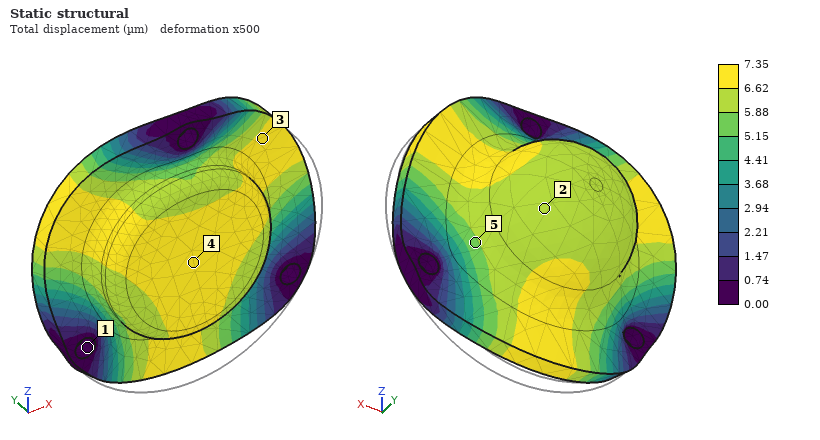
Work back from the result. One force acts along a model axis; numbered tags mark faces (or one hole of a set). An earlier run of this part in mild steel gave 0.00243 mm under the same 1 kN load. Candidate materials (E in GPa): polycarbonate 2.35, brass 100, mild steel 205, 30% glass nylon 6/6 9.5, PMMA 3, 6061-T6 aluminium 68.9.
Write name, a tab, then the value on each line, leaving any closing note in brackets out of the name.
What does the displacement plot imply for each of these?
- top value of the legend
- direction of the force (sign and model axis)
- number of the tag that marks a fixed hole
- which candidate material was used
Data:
top value of the legend	7.35 µm
direction of the force	+Y
number of the tag that marks a fixed hole	1
which candidate material was used	6061-T6 aluminium
